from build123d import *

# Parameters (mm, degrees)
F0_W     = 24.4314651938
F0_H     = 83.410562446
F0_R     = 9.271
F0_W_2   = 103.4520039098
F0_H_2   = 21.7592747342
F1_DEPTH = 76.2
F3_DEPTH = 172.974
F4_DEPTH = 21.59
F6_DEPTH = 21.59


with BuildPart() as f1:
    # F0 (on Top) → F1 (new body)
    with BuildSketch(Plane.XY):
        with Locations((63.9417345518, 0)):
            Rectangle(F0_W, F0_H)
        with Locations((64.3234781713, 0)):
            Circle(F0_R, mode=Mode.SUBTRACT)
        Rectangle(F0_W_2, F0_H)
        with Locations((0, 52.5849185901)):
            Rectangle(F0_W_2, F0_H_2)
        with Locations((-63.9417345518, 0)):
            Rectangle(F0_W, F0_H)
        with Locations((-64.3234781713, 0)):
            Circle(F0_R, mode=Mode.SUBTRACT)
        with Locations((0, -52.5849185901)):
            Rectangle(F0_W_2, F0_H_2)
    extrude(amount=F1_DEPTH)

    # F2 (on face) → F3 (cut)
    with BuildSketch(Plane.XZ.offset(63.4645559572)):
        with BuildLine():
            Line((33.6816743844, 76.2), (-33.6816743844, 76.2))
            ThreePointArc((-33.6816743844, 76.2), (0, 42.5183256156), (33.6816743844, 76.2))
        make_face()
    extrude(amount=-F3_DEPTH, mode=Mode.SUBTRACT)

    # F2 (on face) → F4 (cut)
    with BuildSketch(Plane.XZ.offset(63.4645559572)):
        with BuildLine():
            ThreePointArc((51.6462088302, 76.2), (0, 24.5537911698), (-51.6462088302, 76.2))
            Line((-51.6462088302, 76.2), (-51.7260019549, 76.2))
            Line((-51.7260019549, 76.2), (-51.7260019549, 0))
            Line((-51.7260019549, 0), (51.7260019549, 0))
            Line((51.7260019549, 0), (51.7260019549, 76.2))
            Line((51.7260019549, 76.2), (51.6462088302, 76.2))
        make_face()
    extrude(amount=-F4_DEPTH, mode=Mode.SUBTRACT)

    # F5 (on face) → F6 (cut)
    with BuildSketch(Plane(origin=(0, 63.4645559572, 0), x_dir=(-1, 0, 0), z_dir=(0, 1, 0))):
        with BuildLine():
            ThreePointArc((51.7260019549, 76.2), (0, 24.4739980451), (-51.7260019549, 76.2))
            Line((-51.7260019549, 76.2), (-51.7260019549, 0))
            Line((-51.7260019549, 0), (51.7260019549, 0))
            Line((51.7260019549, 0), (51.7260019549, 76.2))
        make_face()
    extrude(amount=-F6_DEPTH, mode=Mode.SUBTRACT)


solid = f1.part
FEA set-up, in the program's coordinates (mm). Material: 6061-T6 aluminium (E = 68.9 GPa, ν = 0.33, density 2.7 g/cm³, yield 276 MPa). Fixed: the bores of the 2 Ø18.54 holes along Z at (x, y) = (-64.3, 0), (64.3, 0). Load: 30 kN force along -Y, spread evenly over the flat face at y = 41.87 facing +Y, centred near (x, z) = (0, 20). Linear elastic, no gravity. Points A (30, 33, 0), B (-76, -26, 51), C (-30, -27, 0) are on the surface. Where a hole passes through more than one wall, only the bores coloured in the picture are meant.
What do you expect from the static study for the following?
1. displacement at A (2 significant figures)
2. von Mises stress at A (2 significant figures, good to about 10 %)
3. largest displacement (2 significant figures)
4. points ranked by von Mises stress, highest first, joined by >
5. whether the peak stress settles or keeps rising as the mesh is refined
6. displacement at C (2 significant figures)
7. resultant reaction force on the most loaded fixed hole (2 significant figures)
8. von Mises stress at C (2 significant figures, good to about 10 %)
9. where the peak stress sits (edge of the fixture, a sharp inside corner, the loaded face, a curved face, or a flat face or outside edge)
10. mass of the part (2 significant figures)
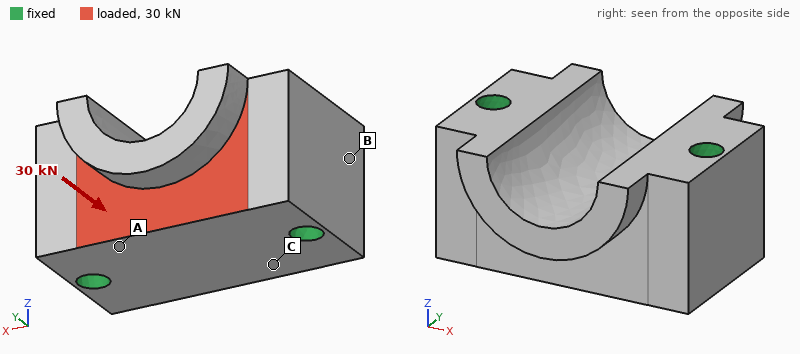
11 µm
7.9 MPa
14 µm
A > C > B
keeps rising
6.4 µm
15 kN
4.8 MPa
edge of the fixture
2.4 kg
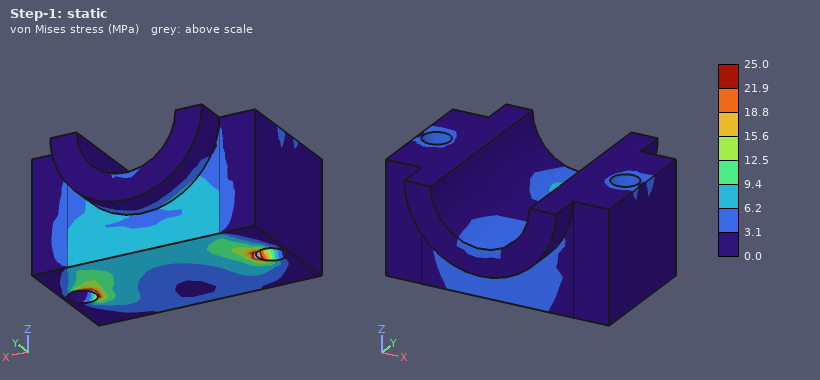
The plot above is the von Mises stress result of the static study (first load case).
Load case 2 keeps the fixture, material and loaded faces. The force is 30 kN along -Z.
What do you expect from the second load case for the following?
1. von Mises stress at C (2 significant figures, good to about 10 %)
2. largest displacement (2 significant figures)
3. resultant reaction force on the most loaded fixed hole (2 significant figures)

4.3 MPa
27 µm
15 kN
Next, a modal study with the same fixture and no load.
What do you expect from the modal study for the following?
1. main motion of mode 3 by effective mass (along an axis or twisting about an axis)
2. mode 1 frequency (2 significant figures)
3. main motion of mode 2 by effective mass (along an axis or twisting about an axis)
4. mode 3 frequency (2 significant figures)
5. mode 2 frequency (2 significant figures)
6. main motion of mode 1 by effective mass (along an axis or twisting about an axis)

along Y
8200 Hz
along Z
9600 Hz
8700 Hz
along Y
